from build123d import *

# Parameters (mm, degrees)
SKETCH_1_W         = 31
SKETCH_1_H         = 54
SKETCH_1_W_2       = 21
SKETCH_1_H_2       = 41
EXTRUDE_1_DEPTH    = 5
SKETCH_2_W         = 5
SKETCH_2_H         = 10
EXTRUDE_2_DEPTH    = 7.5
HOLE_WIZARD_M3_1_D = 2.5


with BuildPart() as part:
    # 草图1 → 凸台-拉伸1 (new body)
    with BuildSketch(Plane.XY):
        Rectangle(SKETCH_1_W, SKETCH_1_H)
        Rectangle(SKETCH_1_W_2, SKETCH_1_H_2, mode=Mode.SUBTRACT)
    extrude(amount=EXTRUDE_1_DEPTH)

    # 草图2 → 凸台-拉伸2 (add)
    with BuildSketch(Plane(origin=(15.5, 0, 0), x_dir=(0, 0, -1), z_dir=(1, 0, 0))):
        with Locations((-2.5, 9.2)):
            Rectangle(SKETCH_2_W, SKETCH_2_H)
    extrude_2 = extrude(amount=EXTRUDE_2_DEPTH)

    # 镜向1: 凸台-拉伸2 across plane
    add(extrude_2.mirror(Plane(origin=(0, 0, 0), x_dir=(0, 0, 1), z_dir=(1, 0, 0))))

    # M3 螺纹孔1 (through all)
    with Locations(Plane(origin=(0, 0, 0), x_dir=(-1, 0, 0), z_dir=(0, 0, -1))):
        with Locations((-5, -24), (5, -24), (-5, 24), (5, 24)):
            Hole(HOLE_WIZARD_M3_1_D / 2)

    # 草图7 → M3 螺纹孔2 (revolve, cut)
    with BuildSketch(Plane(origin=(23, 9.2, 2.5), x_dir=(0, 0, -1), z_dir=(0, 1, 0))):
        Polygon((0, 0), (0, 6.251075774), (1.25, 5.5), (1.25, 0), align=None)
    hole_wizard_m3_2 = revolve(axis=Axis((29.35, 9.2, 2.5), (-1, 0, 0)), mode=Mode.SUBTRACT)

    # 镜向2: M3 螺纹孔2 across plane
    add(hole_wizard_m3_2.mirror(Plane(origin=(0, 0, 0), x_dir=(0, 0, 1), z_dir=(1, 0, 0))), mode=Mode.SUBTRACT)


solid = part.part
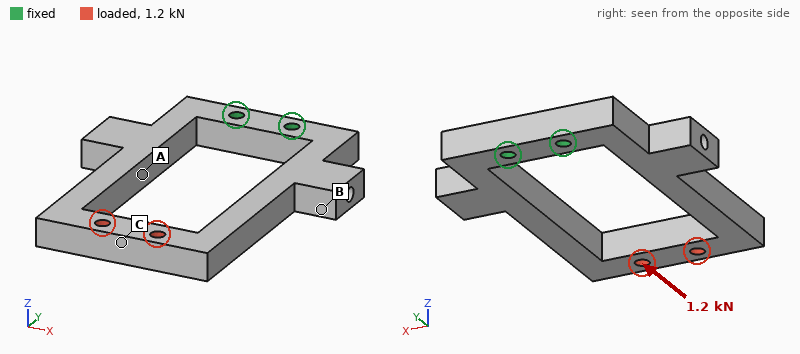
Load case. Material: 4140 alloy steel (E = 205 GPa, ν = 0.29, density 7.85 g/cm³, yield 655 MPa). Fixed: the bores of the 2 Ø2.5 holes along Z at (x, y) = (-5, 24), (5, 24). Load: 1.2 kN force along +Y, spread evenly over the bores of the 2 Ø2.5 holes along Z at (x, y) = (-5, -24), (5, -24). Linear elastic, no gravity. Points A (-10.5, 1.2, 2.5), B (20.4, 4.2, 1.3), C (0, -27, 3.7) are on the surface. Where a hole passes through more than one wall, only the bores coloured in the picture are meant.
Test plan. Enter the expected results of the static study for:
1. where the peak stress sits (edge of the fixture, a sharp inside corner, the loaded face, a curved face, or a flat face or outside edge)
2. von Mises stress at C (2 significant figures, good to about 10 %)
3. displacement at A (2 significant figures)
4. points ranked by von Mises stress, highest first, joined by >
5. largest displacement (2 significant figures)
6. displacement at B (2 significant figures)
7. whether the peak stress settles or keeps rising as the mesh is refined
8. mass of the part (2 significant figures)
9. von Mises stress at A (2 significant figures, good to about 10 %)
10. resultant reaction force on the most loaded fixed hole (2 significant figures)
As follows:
edge of the fixture
110 MPa
18 µm
C > A > B
27 µm
20 µm
keeps rising
37 g
54 MPa
610 N
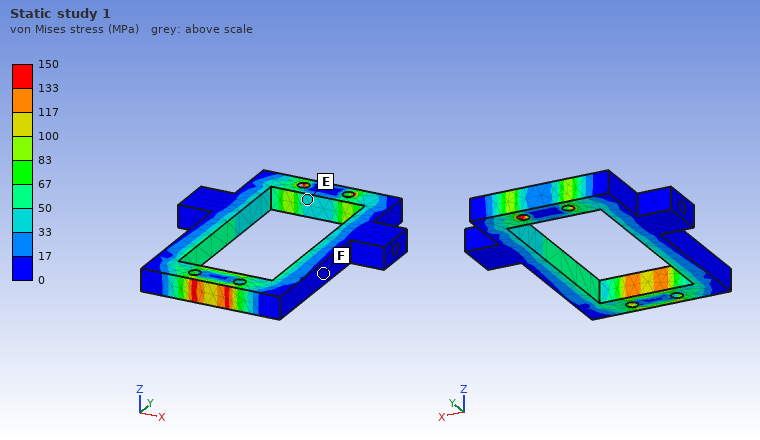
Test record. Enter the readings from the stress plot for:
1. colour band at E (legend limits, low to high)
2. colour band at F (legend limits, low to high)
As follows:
33 to 50 MPa
0 to 17 MPa
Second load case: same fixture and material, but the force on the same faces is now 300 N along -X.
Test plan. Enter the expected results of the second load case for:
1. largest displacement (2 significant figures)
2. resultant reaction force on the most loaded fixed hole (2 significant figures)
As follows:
0.19 mm
710 N
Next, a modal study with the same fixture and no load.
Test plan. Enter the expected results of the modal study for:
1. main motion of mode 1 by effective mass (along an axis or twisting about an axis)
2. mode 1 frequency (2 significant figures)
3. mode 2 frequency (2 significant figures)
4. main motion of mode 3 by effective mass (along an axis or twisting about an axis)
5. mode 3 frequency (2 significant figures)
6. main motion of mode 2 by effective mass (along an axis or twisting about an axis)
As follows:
along Z
1000 Hz
1700 Hz
twisting about Y
2700 Hz
along X
